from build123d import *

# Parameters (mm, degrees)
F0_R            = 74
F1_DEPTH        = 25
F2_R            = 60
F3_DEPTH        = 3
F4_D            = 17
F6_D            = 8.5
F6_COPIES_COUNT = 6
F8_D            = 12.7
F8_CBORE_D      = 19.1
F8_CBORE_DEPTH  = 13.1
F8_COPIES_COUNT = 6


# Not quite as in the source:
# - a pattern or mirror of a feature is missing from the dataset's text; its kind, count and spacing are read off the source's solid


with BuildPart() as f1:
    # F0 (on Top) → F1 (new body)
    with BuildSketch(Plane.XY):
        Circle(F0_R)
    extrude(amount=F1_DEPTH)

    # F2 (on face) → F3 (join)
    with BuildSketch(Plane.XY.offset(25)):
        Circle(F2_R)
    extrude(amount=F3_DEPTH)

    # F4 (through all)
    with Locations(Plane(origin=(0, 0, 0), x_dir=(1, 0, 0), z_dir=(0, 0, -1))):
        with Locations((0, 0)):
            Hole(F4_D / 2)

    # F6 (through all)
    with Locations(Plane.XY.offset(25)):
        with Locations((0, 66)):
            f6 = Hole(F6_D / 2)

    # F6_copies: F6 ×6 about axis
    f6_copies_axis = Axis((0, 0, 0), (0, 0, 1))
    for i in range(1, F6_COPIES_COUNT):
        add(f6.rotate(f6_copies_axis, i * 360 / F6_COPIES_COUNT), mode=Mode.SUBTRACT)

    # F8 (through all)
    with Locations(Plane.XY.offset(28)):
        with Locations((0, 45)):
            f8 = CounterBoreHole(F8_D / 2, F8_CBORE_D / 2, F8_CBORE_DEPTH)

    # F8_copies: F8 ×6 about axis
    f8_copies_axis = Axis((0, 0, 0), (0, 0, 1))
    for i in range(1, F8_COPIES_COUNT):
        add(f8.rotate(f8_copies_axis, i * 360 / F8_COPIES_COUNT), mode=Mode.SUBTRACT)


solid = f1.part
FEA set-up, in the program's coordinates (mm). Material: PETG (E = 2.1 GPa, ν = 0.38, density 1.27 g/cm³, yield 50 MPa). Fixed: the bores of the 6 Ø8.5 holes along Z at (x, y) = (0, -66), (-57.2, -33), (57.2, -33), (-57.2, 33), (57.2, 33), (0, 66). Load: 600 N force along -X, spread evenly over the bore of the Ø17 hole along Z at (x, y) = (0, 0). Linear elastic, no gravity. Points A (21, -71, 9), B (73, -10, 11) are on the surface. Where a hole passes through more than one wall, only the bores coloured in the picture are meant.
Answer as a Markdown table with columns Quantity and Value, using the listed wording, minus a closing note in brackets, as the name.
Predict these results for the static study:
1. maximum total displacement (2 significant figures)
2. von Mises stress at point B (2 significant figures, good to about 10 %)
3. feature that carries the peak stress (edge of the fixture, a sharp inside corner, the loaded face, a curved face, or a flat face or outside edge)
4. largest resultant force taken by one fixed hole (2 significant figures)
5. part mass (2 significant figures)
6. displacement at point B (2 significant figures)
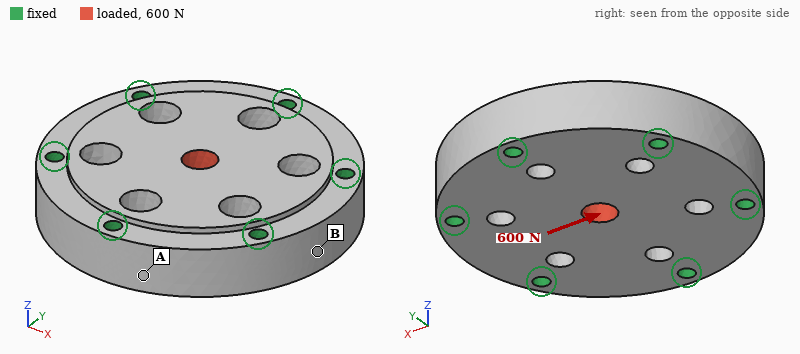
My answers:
| Quantity | Value |
|---|---|
| maximum total displacement | 9.1 µm |
| von Mises stress at point B | 0.17 MPa |
| feature that carries the peak stress | the loaded face |
| largest resultant force taken by one fixed hole | 130 N |
| part mass | 530 g |
| displacement at point B | 3.3 µm |
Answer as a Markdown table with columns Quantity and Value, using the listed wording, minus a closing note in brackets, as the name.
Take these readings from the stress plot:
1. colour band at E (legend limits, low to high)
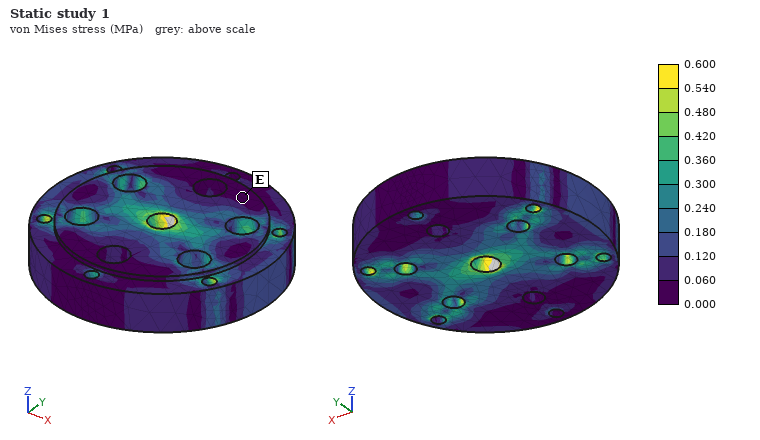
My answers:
| Quantity | Value |
|---|---|
| colour band at E | 0.000 to 0.060 MPa |
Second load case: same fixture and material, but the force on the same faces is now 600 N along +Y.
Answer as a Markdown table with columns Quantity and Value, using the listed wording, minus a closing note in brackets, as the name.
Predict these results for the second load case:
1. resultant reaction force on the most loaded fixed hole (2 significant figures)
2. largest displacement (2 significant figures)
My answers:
| Quantity | Value |
|---|---|
| resultant reaction force on the most loaded fixed hole | 150 N |
| largest displacement | 9.1 µm |
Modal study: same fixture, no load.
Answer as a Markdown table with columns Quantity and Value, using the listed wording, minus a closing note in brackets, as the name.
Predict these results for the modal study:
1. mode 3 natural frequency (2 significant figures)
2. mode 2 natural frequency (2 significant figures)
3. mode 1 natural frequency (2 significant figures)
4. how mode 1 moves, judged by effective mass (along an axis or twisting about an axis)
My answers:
| Quantity | Value |
|---|---|
| mode 3 natural frequency | 3500 Hz |
| mode 2 natural frequency | 3500 Hz |
| mode 1 natural frequency | 2100 Hz |
| how mode 1 moves, judged by effective mass | along Z |
